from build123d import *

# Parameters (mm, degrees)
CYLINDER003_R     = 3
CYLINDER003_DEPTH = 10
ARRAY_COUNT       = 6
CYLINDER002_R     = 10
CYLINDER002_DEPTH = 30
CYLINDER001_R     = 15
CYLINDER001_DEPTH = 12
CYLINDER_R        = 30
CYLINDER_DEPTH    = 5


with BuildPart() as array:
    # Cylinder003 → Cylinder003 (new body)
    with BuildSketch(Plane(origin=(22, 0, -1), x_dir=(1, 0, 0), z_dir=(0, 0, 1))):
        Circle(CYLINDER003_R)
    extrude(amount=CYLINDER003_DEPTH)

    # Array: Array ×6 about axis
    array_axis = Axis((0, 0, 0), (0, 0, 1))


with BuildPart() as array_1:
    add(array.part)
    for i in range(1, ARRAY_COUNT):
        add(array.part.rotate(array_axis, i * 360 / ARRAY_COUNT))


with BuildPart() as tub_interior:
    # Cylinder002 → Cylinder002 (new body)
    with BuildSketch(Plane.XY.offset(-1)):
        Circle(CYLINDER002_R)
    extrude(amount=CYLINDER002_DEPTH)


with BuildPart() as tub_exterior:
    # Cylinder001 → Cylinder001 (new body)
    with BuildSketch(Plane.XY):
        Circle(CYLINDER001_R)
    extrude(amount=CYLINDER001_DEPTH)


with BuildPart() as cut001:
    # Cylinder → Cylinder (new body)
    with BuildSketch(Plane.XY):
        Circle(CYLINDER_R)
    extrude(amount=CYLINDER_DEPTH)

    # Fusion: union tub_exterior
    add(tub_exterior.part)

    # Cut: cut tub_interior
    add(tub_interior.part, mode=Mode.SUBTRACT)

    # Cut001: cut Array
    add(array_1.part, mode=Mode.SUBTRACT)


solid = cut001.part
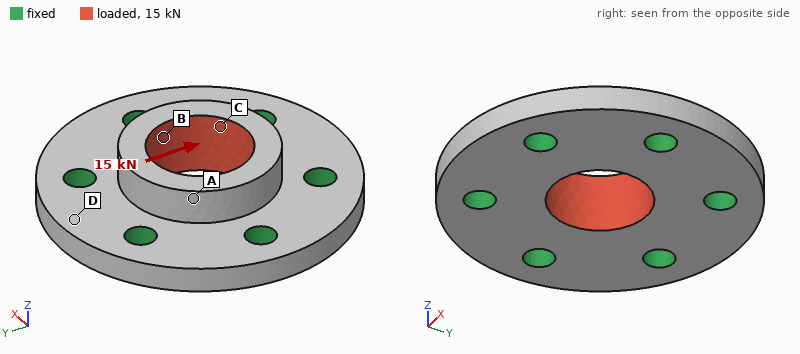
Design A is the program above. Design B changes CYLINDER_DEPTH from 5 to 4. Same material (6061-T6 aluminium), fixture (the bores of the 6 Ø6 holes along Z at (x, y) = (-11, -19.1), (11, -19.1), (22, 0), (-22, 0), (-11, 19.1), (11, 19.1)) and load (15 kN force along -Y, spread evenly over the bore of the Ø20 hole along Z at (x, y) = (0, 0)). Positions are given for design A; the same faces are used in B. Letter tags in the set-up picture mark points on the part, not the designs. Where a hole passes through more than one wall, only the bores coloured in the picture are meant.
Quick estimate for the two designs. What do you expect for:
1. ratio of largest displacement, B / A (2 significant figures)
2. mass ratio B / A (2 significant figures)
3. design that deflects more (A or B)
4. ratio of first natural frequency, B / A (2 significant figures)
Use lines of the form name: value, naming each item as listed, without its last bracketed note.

ratio of largest displacement, B / A: 1.3
mass ratio B / A: 0.87
design that deflects more: B
ratio of first natural frequency, B / A: 0.87
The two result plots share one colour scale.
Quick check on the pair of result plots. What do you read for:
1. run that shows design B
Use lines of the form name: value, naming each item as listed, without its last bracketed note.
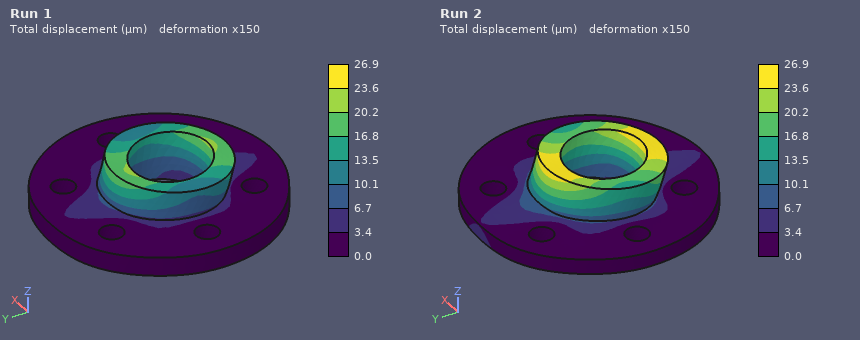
run that shows design B: Run 2
